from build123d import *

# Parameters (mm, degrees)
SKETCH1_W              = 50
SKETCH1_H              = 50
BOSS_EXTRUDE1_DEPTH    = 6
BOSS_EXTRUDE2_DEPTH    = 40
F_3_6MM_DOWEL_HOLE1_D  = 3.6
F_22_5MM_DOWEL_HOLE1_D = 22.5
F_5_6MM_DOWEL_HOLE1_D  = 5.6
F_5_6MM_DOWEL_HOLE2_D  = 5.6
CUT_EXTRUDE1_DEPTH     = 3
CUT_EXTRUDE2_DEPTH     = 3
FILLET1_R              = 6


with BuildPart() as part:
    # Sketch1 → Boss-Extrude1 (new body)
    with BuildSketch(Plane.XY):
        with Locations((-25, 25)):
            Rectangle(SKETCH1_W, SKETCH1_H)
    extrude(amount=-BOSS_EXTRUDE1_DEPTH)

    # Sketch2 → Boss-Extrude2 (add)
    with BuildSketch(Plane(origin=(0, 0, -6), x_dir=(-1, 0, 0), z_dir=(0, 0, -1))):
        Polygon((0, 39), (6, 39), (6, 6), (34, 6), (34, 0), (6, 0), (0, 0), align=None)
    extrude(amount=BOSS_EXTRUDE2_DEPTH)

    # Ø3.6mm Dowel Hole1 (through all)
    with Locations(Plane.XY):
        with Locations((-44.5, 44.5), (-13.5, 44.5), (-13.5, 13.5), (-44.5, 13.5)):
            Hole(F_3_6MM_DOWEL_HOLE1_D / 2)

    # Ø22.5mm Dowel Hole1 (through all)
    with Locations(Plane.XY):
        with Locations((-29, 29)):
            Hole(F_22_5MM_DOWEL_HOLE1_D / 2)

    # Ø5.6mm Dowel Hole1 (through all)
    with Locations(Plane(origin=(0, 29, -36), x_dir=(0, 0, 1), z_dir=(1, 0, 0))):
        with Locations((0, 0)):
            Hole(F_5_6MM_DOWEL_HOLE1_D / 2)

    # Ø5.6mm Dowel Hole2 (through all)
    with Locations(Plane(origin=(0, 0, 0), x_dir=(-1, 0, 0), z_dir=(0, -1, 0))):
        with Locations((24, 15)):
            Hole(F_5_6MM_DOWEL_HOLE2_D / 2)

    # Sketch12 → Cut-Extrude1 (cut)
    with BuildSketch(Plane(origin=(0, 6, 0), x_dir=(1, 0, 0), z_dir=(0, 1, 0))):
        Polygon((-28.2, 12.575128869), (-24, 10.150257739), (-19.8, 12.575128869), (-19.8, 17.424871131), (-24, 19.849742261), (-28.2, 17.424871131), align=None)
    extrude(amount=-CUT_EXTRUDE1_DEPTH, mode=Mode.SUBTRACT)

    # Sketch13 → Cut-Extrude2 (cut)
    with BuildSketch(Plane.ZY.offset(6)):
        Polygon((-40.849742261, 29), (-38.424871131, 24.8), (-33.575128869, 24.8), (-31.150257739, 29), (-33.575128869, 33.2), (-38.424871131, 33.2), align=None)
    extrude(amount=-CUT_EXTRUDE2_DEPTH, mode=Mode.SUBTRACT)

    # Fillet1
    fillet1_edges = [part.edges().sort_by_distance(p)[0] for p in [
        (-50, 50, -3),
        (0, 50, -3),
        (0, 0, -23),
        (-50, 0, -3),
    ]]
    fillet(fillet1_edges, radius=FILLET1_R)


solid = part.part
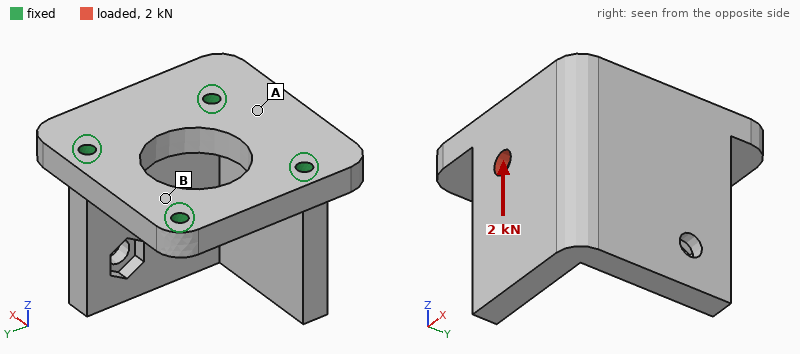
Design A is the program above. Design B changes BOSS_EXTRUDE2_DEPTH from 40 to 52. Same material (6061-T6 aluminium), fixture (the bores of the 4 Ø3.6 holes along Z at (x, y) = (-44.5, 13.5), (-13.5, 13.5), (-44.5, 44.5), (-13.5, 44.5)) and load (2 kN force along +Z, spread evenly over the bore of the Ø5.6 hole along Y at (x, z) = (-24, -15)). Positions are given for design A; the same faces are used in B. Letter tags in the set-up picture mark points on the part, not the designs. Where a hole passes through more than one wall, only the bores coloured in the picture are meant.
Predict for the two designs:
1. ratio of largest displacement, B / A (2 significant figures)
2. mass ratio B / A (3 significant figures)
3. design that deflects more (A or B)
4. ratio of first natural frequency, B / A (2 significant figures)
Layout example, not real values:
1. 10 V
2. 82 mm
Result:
1. 1.1
2. 1.17
3. B
4. 0.70
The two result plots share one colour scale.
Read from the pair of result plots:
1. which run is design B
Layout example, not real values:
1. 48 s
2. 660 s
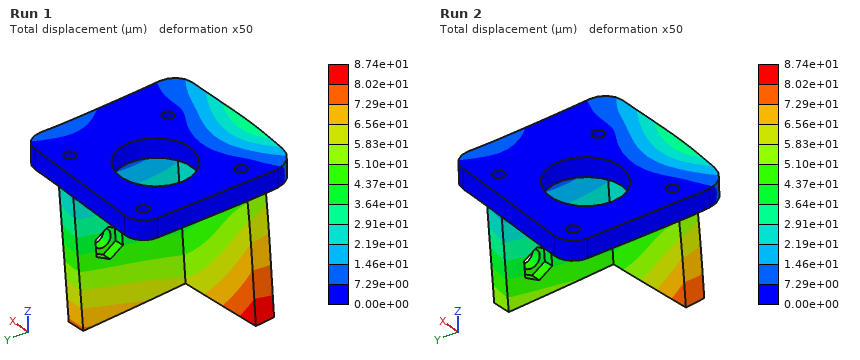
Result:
1. Run 1
